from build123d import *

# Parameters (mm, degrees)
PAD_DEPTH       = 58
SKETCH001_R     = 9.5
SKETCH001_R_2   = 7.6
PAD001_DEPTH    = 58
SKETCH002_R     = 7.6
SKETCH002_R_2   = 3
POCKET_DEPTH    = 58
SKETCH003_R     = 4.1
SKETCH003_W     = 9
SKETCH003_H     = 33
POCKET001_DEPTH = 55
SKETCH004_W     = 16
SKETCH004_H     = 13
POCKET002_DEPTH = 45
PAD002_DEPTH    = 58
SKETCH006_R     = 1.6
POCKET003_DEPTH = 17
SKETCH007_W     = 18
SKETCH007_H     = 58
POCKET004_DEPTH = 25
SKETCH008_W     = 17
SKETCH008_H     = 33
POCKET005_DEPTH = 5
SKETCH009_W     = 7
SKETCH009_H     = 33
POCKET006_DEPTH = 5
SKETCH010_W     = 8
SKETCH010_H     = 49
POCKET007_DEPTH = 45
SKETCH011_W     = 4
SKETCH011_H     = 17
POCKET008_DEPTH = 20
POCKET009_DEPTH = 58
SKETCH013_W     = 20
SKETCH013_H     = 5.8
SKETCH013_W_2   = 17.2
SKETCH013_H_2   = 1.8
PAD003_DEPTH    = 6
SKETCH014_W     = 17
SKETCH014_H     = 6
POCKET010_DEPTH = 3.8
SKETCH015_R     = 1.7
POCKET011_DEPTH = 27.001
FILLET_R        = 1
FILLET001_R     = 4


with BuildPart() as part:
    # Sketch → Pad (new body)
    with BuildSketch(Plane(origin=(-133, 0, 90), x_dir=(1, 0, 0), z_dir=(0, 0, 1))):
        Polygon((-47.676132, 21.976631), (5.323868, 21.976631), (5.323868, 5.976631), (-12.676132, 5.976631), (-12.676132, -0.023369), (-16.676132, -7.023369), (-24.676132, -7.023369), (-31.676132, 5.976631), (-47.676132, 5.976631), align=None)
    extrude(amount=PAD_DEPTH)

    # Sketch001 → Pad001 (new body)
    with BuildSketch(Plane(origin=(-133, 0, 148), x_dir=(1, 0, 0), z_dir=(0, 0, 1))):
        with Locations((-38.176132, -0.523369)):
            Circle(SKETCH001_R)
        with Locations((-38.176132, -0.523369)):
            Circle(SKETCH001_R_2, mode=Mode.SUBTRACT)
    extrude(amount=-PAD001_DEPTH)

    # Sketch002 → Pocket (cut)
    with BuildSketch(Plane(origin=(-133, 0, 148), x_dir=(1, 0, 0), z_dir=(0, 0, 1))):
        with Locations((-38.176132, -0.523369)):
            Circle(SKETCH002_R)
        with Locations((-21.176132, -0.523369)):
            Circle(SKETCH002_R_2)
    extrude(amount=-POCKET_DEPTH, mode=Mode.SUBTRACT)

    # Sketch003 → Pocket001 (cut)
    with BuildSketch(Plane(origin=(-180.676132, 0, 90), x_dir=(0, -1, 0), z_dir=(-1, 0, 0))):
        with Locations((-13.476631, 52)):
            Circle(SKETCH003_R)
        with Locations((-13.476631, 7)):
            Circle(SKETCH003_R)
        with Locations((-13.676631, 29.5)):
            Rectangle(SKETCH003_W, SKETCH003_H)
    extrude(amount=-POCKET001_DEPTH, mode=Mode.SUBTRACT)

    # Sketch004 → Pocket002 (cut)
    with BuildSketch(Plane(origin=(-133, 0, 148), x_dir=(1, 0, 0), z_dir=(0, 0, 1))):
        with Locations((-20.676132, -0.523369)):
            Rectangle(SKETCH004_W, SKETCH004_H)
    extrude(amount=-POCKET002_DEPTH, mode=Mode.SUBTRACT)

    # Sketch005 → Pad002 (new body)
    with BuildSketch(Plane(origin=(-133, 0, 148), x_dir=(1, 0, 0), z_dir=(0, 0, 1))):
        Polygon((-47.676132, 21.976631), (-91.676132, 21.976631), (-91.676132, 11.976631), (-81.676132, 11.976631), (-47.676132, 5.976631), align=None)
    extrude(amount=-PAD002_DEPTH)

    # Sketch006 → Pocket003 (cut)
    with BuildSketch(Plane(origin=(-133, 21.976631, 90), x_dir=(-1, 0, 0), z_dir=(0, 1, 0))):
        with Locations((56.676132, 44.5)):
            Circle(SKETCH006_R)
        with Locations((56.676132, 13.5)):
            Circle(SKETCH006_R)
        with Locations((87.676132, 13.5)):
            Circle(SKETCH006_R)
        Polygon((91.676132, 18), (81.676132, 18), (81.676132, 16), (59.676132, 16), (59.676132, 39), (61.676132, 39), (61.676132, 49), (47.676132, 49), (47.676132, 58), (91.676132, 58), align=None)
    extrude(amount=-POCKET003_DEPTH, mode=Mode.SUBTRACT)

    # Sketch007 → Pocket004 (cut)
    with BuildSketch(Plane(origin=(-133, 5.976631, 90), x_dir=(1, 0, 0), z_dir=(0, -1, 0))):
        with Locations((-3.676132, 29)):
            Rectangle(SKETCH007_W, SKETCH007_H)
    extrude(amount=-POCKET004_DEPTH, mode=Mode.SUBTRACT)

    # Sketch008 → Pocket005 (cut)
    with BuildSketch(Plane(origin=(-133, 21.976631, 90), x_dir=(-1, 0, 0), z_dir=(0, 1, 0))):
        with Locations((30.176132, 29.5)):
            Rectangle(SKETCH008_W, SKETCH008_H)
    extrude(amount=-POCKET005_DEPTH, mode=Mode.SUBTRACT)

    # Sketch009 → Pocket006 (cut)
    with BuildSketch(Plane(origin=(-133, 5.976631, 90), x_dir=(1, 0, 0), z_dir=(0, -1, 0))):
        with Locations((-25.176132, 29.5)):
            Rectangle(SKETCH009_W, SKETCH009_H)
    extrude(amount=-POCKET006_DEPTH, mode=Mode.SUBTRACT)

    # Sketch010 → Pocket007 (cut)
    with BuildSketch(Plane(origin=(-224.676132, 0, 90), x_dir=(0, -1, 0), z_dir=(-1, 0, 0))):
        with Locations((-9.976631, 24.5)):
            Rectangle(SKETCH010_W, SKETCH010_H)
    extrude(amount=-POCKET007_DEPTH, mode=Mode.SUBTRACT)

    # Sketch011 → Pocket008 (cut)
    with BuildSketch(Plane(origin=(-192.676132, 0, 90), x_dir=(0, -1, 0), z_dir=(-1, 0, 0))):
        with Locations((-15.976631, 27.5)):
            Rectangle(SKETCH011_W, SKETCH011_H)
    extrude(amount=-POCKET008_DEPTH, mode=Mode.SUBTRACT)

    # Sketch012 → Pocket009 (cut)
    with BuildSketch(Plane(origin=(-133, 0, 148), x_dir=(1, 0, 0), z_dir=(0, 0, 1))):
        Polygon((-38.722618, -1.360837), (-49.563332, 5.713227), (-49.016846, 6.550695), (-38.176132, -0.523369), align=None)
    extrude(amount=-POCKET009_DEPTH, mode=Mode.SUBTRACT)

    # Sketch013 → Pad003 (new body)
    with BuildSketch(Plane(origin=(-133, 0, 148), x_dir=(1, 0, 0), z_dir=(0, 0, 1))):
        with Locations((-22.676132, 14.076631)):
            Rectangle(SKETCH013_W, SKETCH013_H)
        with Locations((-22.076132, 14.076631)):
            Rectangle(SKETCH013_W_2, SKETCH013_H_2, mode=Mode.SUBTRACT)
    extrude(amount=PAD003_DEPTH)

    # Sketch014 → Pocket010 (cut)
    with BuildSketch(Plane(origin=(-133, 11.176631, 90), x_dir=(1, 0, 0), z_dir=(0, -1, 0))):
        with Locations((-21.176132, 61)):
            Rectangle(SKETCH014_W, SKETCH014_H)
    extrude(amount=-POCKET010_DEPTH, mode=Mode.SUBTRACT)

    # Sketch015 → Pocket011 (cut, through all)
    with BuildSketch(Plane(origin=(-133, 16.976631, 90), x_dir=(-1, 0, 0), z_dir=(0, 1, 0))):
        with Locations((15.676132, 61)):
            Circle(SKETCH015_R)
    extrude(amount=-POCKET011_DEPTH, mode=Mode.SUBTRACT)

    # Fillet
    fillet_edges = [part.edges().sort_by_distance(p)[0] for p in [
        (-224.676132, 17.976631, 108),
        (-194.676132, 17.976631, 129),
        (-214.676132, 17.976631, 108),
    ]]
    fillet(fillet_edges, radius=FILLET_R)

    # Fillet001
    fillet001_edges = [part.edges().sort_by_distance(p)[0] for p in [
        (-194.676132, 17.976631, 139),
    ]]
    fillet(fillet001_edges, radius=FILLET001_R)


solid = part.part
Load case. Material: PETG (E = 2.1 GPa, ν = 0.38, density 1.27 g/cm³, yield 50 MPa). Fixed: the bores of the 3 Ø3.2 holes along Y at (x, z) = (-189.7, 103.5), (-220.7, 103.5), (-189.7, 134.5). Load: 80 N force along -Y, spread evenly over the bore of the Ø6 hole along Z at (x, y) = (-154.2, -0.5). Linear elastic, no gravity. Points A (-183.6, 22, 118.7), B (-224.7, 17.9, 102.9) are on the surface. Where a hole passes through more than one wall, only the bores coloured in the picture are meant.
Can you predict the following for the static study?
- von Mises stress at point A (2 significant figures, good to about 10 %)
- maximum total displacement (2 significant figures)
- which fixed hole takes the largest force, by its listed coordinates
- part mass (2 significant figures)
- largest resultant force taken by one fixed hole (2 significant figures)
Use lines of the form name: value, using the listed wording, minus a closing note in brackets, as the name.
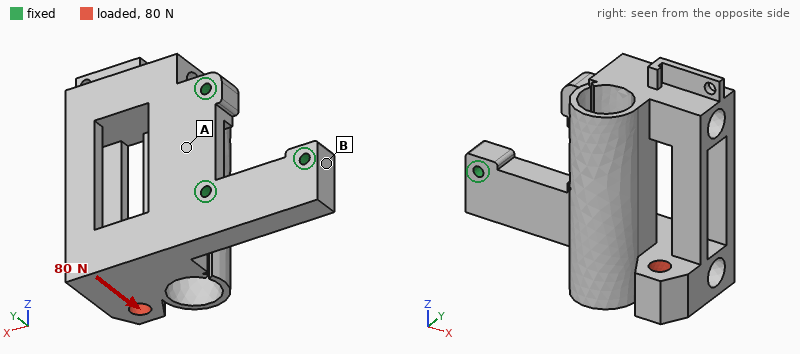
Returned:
von Mises stress at point A: 2.4 MPa
maximum total displacement: 1.1 mm
which fixed hole takes the largest force, by its listed coordinates: (-189.7, 103.5)
part mass: 38 g
largest resultant force taken by one fixed hole: 110 N
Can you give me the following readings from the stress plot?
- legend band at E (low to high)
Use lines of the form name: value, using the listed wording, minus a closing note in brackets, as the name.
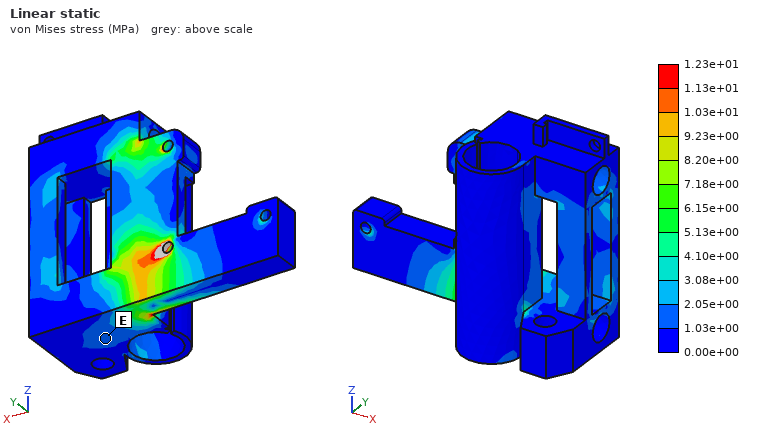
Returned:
legend band at E: 1.03e+00 to 2.05e+00 MPa
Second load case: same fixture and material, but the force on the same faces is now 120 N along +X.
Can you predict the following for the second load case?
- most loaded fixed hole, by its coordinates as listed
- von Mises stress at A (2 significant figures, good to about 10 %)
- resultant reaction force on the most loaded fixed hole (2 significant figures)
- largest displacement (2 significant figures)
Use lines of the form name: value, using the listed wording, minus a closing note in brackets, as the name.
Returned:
most loaded fixed hole, by its coordinates as listed: (-189.7, 103.5)
von Mises stress at A: 2.0 MPa
resultant reaction force on the most loaded fixed hole: 91 N
largest displacement: 1.1 mm
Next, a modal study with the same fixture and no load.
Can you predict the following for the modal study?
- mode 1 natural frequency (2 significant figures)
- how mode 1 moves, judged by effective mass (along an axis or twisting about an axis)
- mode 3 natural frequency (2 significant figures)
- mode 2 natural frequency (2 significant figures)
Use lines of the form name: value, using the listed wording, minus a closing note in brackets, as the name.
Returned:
mode 1 natural frequency: 400 Hz
how mode 1 moves, judged by effective mass: along Y
mode 3 natural frequency: 620 Hz
mode 2 natural frequency: 500 Hz
